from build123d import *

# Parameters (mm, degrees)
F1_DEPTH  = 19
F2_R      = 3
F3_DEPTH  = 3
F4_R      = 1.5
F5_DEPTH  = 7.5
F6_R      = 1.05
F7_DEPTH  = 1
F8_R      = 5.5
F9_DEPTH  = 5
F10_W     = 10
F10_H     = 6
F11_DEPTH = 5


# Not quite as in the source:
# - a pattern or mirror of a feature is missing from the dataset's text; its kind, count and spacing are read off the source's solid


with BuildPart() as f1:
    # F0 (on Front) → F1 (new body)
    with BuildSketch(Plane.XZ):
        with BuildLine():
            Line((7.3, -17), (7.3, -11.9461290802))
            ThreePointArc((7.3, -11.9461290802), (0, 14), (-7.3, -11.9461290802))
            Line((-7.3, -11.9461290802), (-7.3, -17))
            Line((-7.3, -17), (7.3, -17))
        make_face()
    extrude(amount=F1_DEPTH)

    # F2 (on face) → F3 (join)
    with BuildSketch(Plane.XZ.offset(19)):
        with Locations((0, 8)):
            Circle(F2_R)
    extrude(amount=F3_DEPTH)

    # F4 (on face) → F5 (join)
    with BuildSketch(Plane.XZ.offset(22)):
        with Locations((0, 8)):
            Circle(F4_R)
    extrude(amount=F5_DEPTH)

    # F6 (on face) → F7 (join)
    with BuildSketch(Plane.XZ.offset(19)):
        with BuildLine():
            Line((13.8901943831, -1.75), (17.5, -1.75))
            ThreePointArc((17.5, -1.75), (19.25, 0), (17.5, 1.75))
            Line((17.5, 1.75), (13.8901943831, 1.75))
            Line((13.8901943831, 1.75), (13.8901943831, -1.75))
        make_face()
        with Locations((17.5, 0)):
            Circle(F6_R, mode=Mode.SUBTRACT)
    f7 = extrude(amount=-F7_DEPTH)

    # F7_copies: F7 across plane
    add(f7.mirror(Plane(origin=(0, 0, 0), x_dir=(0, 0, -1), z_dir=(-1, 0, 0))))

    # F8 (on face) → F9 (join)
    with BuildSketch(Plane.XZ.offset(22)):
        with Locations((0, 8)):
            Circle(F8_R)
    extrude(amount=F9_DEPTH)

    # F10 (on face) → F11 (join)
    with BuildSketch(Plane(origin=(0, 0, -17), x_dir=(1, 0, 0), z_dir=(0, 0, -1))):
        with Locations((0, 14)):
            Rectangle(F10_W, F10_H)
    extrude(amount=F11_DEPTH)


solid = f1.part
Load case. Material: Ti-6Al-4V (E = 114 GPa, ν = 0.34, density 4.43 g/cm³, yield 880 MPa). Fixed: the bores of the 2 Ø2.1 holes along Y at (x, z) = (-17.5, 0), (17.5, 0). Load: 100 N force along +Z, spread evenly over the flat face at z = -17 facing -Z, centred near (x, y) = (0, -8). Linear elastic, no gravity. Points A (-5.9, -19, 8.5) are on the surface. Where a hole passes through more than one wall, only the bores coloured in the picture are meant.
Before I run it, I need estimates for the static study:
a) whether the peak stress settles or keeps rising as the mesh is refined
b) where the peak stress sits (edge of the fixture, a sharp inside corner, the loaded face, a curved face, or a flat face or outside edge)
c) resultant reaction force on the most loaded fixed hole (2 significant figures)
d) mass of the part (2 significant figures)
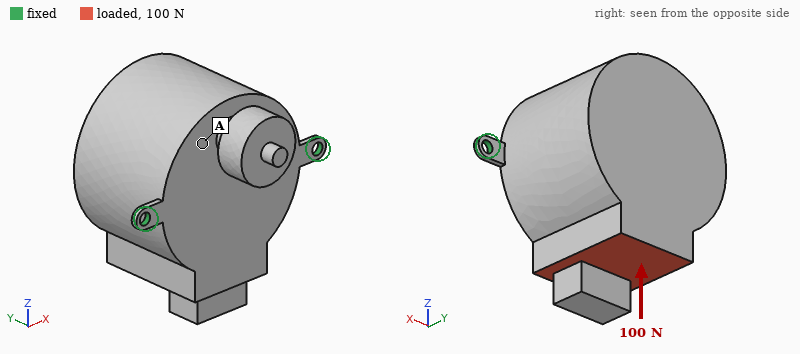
keeps rising
edge of the fixture
50 N
60 g
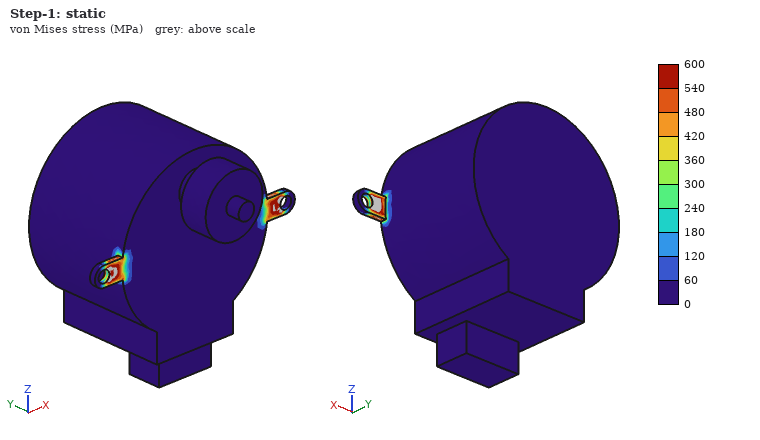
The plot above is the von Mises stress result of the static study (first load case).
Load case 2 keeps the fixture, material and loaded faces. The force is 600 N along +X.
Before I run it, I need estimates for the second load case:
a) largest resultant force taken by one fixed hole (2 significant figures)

490 N
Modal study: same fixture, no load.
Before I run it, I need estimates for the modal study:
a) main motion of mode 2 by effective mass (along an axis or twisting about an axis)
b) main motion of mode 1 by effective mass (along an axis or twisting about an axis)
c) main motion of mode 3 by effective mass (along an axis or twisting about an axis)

along Y
along Z
along X
